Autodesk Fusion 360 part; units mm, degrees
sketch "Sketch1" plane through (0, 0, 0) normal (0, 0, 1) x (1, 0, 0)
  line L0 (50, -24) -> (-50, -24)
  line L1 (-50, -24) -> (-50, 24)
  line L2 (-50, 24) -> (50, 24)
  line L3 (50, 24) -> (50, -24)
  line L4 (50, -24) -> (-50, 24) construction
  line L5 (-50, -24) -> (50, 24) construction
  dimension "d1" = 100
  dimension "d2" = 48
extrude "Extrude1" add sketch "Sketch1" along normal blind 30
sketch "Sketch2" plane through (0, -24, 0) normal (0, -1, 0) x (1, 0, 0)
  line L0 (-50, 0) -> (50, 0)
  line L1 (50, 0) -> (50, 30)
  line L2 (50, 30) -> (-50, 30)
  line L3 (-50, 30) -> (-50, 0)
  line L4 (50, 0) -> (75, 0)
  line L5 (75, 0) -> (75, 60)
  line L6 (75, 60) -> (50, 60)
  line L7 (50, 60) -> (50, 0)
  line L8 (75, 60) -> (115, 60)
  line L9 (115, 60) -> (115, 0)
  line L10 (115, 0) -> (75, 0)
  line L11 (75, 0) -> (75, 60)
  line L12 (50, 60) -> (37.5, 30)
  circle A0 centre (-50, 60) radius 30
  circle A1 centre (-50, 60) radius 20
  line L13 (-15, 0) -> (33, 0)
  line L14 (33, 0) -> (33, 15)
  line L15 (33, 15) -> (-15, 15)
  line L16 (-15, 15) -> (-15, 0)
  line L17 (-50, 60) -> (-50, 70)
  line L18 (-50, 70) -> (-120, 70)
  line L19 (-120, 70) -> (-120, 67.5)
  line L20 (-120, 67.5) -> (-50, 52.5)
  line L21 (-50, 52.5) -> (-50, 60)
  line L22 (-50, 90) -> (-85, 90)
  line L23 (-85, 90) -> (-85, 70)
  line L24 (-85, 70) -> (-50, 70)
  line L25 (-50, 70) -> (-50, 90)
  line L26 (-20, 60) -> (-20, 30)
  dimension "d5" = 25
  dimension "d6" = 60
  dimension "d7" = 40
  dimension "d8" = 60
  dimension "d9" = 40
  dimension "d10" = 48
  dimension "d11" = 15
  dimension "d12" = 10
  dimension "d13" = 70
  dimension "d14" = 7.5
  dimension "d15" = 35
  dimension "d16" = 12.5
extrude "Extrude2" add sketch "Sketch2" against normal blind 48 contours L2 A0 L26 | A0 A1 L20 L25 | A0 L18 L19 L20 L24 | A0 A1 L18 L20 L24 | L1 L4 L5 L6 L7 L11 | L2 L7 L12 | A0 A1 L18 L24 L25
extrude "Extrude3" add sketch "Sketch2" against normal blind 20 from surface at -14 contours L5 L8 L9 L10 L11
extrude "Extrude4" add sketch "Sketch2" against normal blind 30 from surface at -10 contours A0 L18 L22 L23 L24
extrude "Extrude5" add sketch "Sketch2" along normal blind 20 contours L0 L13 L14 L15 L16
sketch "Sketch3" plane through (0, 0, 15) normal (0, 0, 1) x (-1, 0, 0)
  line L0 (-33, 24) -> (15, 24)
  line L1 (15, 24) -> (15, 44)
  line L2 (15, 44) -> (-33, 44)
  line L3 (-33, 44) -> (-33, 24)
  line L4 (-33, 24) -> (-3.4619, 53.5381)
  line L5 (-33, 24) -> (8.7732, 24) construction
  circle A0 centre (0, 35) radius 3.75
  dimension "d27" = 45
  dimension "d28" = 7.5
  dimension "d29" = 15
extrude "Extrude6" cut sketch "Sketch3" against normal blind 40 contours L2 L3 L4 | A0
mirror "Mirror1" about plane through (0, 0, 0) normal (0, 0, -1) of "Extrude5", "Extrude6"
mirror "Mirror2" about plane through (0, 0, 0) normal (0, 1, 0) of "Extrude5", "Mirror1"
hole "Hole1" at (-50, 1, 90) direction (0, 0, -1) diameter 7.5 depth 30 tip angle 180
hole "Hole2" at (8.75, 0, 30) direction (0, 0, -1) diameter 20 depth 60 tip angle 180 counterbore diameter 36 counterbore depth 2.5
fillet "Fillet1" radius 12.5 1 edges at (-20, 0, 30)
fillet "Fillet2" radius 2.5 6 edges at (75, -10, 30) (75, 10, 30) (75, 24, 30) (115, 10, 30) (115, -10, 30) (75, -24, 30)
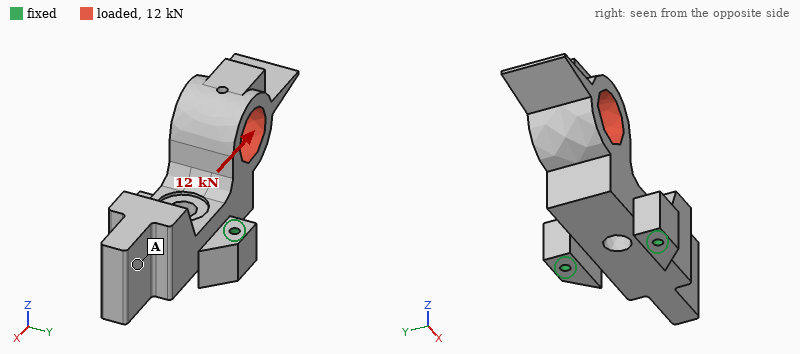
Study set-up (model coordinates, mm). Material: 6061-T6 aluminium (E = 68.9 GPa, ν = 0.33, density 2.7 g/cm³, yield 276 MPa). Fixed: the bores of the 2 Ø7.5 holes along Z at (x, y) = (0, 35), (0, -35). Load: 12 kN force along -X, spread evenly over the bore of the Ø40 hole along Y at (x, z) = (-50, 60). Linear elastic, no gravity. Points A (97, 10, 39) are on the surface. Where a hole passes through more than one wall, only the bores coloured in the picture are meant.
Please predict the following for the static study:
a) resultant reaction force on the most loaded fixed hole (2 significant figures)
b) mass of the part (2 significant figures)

6.5 kN
1.1 kg
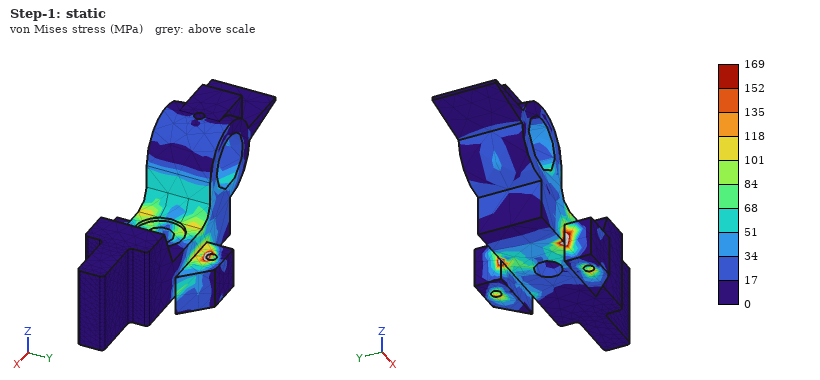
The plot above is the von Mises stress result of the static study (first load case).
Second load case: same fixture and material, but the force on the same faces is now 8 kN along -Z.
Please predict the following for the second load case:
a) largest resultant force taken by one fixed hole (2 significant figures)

5.4 kN
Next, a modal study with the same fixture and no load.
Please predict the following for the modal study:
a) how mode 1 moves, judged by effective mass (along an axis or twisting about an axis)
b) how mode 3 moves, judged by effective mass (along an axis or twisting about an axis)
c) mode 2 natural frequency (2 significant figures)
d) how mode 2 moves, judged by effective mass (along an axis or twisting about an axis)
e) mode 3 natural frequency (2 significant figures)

along X
along Y
1600 Hz
along Z
2200 Hz
